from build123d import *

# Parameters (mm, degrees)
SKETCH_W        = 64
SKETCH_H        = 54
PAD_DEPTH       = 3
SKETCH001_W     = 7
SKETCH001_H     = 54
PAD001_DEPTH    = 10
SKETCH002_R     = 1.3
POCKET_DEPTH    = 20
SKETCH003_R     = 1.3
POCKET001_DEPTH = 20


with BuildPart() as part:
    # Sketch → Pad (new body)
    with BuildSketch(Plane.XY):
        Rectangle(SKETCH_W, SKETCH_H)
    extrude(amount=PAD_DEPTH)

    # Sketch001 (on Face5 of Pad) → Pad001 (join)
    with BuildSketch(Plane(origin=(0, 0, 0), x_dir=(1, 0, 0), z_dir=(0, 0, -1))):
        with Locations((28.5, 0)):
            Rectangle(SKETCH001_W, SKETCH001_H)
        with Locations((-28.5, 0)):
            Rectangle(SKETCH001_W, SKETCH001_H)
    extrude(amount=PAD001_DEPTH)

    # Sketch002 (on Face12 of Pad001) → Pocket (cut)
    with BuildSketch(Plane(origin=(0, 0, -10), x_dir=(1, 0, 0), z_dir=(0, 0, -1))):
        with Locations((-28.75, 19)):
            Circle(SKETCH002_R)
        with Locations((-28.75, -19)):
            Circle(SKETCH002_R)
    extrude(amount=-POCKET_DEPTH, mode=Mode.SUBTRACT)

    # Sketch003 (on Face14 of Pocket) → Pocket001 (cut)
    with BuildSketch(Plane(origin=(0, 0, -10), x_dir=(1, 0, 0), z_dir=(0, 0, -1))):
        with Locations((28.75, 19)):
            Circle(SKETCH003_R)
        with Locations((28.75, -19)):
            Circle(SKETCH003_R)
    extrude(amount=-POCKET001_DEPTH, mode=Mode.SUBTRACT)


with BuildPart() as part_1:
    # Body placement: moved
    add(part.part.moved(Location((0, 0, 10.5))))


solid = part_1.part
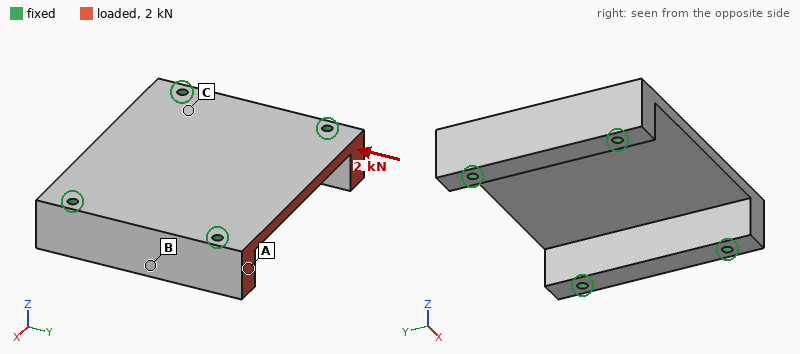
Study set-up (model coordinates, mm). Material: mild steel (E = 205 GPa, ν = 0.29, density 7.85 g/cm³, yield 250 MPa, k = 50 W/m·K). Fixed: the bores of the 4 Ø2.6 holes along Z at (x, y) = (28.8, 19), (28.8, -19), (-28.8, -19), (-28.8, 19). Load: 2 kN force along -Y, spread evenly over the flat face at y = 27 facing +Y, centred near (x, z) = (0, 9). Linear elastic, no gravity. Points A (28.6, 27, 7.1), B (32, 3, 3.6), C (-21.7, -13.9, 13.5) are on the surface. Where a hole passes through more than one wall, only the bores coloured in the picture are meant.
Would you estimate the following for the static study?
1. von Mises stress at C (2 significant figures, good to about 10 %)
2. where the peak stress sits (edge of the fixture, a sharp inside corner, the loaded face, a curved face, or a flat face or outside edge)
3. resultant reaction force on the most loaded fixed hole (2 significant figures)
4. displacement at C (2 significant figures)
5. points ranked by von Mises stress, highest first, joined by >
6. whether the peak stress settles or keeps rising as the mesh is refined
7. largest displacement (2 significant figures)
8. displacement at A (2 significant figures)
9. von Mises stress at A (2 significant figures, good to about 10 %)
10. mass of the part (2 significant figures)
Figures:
4.5 MPa
edge of the fixture
800 N
0.21 µm
A > C > B
keeps rising
1.3 µm
0.32 µm
6.9 MPa
140 g
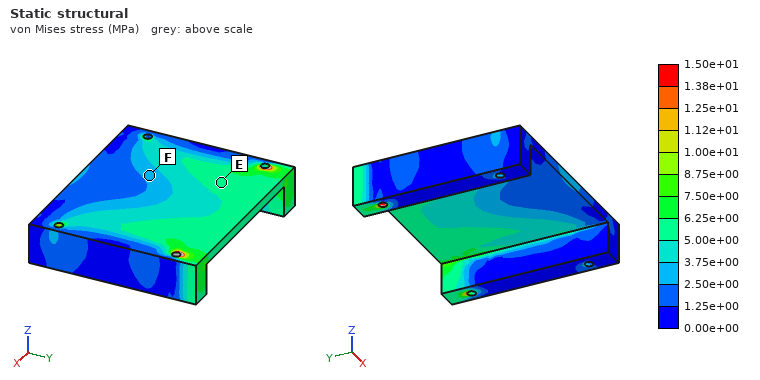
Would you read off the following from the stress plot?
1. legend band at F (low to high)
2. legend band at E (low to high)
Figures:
2.50e+00 to 3.75e+00 MPa
5.00e+00 to 6.25e+00 MPa
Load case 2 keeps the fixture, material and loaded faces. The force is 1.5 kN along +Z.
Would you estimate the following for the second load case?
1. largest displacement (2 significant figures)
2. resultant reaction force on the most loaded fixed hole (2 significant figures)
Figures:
54 µm
800 N
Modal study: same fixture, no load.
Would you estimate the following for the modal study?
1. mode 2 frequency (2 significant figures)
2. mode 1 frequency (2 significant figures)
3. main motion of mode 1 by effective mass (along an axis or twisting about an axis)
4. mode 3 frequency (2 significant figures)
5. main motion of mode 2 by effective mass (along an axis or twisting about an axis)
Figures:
6600 Hz
5500 Hz
along Z
10 kHz
twisting about X
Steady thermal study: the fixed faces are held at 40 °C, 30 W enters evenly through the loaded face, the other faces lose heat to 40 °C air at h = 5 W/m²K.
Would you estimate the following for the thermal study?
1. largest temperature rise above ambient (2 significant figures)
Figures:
40 K
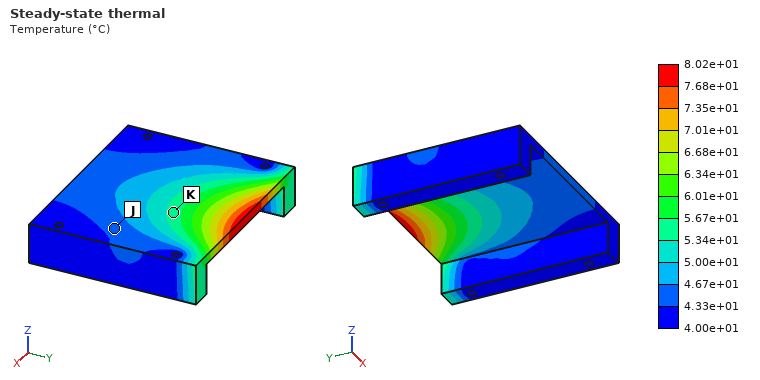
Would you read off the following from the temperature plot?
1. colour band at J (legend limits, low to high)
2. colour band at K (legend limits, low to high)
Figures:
4.33e+01 to 4.67e+01 °C
5.34e+01 to 5.67e+01 °C
